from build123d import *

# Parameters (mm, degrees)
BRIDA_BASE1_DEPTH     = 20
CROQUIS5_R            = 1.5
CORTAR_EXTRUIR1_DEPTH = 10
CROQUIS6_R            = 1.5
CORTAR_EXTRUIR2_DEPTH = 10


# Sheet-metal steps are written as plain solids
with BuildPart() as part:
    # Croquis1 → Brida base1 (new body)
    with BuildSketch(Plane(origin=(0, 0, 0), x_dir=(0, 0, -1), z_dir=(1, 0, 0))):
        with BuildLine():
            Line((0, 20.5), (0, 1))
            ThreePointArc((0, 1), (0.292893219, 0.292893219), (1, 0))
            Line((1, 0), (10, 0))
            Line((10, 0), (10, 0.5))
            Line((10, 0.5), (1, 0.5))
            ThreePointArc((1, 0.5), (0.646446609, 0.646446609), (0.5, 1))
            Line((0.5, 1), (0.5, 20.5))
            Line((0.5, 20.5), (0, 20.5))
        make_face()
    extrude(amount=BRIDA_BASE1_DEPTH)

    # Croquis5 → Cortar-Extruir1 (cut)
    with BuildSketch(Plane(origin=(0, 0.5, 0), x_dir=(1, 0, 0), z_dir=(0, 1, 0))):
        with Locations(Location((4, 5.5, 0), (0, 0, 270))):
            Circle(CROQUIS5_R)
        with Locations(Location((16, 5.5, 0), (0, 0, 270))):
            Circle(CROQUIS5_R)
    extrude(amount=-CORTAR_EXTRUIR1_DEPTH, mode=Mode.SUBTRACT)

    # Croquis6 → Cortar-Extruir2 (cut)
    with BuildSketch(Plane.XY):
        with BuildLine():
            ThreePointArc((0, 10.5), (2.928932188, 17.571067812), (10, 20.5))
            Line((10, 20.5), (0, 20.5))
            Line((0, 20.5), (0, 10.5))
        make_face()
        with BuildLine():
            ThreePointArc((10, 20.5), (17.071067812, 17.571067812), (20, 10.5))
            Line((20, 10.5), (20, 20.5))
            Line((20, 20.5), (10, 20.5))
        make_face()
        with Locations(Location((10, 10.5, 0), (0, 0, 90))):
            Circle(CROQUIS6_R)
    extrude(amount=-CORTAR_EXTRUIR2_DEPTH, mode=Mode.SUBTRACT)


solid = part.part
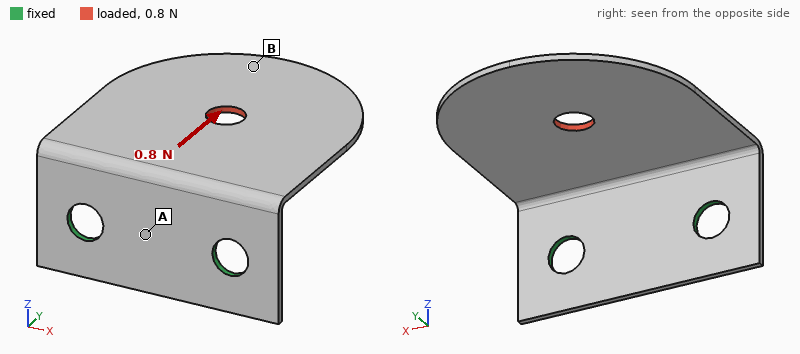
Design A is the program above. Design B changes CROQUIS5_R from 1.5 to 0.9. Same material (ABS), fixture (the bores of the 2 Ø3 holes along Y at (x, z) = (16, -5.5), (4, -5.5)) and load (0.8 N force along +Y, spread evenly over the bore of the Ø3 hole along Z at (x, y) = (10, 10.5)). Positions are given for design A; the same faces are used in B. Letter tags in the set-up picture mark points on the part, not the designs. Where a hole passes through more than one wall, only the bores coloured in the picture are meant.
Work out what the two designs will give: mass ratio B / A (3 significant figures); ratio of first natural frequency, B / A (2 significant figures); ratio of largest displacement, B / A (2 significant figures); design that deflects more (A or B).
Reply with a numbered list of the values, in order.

1. 1.02
2. 0.95
3. 1.4
4. B
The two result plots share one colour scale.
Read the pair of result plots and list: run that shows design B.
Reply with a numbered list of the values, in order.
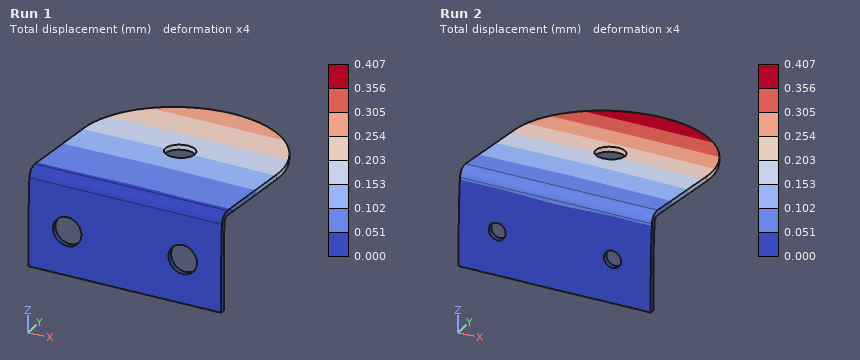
1. Run 2
